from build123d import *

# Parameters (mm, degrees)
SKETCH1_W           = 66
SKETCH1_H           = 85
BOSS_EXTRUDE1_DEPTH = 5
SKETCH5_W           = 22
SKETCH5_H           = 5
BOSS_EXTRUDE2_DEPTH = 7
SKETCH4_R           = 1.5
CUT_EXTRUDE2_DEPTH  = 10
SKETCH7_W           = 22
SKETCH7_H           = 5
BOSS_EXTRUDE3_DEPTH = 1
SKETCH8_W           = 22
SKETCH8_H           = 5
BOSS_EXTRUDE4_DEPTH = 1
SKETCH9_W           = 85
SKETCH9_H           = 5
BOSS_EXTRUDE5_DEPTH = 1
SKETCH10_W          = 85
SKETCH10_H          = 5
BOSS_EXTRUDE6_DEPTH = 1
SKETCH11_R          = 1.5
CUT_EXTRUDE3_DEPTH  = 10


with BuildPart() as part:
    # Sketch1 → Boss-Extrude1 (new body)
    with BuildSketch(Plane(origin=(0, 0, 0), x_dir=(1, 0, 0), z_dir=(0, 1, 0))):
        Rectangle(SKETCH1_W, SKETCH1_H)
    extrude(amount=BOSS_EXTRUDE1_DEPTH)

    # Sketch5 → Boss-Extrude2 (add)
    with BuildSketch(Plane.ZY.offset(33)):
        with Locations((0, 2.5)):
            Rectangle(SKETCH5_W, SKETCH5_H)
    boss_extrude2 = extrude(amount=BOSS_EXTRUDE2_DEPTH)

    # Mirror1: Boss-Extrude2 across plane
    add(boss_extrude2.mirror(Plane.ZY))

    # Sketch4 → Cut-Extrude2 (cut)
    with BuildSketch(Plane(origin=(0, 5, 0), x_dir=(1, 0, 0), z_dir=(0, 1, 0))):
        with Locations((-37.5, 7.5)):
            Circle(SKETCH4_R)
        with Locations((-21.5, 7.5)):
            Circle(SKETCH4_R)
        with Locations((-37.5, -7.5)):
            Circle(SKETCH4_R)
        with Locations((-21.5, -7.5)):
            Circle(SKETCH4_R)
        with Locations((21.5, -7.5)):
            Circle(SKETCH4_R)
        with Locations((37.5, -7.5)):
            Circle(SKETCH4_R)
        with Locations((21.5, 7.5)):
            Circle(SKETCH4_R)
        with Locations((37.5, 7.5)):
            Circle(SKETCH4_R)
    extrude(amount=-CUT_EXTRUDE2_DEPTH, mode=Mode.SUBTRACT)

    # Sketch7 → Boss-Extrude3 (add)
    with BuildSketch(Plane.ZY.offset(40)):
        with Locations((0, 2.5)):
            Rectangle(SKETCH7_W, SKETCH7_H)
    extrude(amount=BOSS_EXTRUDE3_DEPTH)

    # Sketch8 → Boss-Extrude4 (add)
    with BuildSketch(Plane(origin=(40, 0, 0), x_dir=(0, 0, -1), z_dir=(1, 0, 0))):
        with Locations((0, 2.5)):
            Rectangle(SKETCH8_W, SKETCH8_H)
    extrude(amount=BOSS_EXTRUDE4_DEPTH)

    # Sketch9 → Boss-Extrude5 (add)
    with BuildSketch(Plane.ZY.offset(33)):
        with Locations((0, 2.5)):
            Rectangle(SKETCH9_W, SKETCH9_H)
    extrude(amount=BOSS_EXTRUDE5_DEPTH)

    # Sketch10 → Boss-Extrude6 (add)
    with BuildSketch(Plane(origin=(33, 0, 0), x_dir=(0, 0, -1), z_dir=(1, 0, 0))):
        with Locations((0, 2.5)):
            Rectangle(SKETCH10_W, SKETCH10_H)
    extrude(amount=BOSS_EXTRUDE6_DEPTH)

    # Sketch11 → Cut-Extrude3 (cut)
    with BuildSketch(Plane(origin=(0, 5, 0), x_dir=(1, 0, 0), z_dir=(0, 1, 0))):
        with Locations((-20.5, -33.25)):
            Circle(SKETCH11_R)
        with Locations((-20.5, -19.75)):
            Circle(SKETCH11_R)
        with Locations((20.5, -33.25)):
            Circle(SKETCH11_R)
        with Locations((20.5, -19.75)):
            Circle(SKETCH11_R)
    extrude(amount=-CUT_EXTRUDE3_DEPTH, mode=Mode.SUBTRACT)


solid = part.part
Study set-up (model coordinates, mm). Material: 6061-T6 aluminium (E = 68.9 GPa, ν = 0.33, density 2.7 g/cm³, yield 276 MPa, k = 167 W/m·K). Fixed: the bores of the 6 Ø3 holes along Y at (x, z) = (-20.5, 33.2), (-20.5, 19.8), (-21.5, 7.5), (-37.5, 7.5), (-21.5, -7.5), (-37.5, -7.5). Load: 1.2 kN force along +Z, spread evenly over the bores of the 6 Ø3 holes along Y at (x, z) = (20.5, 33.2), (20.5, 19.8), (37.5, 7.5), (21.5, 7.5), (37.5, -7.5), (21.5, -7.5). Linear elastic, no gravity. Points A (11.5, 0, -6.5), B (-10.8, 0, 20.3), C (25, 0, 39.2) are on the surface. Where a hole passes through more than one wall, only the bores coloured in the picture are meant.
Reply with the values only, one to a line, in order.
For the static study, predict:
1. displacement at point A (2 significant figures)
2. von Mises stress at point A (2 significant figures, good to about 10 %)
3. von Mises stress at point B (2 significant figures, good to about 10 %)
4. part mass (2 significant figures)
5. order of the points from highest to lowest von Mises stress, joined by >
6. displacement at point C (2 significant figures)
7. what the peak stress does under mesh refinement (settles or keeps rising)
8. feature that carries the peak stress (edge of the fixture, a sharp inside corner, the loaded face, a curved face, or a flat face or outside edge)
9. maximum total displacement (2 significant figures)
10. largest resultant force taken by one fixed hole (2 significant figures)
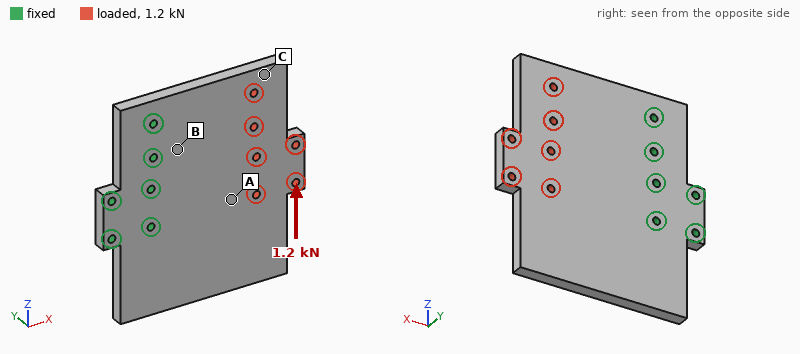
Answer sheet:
12 µm
6.1 MPa
11 MPa
81 g
B > A > C
17 µm
keeps rising
edge of the fixture
22 µm
1.2 kN
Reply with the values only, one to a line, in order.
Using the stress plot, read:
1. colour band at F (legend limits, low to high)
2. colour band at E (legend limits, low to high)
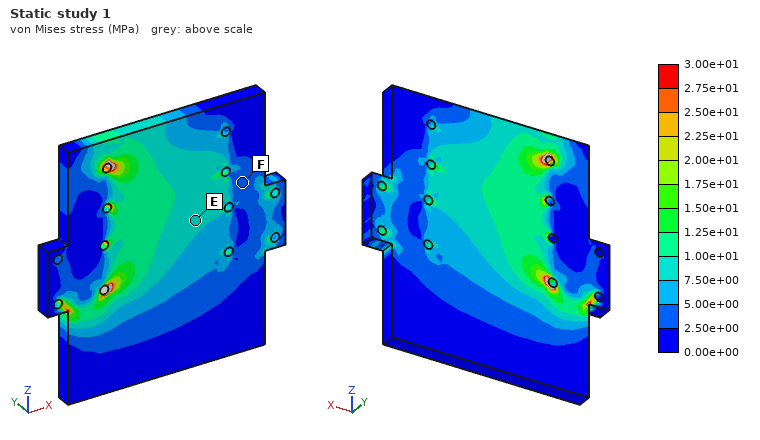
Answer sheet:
2.50e+00 to 5.00e+00 MPa
7.50e+00 to 1.00e+01 MPa
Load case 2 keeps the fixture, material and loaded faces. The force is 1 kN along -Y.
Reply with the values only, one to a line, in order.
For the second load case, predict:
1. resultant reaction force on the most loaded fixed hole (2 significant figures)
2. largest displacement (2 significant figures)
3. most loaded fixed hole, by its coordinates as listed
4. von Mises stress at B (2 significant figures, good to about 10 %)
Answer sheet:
820 N
1.0 mm
(-21.5, -7.5)
120 MPa
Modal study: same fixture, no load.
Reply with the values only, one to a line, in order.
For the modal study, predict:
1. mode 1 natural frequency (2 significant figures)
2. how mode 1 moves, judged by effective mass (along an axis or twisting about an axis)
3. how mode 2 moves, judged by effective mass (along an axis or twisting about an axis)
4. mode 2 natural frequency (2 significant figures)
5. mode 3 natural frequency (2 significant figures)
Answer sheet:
1100 Hz
along Y
twisting about X
1900 Hz
3600 Hz
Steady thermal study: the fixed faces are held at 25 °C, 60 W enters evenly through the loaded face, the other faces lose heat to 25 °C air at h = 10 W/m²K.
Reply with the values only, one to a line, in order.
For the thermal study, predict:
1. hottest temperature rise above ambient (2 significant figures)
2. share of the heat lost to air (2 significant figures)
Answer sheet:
59 K
5.1 %
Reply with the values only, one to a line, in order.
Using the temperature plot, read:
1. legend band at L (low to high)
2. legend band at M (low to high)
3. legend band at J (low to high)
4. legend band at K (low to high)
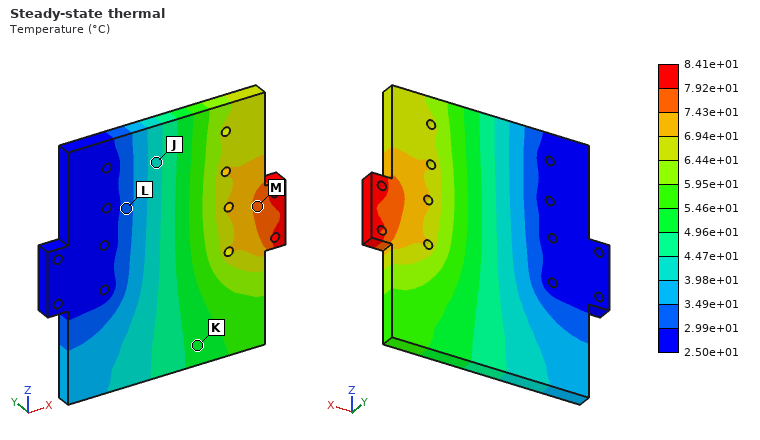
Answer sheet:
2.99e+01 to 3.49e+01 °C
7.43e+01 to 7.92e+01 °C
3.98e+01 to 4.47e+01 °C
4.96e+01 to 5.46e+01 °C
